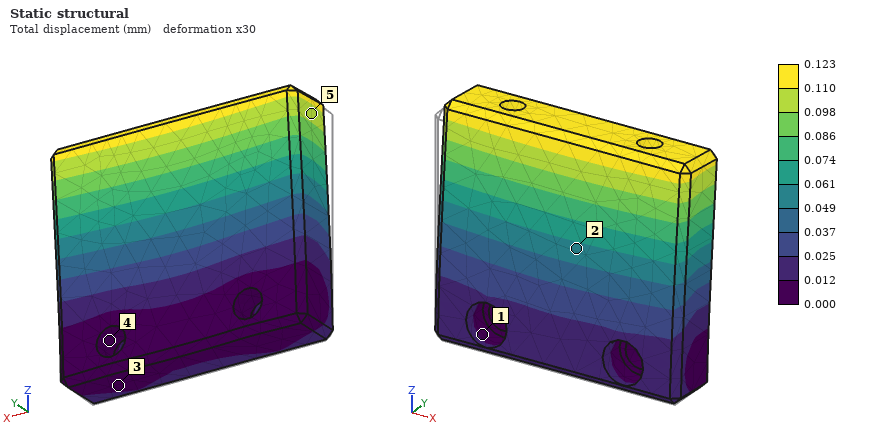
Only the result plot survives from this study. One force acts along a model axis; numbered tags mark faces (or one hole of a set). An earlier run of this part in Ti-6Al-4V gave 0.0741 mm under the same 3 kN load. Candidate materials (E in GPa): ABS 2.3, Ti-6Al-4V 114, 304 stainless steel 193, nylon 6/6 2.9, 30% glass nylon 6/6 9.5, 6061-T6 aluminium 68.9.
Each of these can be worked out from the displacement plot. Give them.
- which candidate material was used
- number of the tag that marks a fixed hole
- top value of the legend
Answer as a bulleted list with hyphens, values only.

- 6061-T6 aluminium
- 4
- 0.123 mm
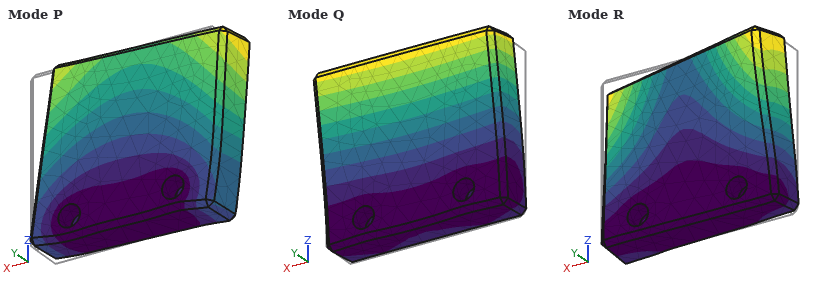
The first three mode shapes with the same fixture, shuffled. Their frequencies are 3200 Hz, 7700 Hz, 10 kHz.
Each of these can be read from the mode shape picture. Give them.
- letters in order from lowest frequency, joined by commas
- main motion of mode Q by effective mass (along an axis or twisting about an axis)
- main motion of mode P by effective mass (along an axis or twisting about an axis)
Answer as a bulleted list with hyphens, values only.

- Q, R, P
- along Y
- along X
